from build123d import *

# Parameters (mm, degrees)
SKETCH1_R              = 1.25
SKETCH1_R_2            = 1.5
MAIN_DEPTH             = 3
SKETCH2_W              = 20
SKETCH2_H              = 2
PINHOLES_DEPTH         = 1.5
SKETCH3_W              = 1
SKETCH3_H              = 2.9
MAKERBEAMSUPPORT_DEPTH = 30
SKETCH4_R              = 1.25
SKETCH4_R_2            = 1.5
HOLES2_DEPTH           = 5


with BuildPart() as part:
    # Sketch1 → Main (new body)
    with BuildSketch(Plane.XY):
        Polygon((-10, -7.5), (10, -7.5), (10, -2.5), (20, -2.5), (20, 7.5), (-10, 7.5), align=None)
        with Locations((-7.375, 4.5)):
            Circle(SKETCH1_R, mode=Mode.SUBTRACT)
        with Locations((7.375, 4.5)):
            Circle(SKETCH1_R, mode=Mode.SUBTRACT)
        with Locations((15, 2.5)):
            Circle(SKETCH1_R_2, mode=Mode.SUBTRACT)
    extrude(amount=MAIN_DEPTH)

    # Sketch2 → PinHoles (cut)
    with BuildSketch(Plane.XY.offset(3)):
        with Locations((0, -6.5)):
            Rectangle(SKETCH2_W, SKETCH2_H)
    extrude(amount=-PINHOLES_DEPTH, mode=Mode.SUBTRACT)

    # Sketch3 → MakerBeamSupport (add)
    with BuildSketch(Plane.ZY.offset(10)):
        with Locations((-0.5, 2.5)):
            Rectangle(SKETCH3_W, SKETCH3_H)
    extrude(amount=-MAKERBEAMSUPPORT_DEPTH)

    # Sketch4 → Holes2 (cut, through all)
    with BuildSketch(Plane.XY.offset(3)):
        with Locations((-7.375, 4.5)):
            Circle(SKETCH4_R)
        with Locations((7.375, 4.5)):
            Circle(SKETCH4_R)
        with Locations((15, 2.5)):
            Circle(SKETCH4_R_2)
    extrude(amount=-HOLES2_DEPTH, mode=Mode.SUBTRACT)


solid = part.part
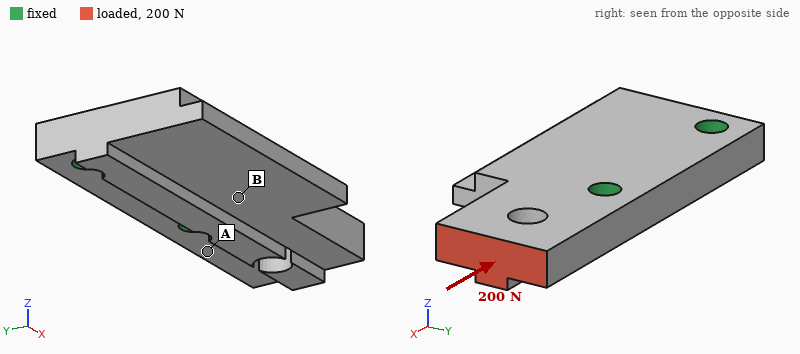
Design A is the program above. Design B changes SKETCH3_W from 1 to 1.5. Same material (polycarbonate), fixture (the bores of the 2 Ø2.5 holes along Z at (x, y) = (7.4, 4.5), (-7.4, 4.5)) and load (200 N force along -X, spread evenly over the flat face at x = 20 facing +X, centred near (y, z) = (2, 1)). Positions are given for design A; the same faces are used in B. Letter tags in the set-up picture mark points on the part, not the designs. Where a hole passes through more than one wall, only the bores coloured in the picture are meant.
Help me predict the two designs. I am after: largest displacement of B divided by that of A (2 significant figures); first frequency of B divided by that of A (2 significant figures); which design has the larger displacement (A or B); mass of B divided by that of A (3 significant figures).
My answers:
1.1
1.0
B
1.02
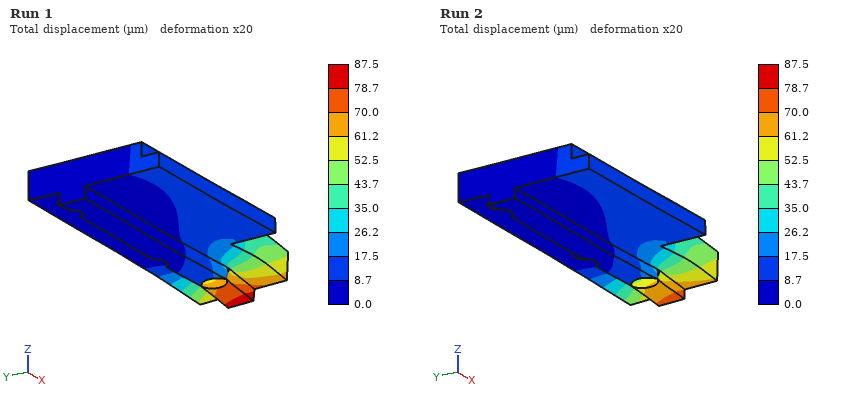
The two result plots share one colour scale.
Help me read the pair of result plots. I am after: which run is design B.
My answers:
Run 1
